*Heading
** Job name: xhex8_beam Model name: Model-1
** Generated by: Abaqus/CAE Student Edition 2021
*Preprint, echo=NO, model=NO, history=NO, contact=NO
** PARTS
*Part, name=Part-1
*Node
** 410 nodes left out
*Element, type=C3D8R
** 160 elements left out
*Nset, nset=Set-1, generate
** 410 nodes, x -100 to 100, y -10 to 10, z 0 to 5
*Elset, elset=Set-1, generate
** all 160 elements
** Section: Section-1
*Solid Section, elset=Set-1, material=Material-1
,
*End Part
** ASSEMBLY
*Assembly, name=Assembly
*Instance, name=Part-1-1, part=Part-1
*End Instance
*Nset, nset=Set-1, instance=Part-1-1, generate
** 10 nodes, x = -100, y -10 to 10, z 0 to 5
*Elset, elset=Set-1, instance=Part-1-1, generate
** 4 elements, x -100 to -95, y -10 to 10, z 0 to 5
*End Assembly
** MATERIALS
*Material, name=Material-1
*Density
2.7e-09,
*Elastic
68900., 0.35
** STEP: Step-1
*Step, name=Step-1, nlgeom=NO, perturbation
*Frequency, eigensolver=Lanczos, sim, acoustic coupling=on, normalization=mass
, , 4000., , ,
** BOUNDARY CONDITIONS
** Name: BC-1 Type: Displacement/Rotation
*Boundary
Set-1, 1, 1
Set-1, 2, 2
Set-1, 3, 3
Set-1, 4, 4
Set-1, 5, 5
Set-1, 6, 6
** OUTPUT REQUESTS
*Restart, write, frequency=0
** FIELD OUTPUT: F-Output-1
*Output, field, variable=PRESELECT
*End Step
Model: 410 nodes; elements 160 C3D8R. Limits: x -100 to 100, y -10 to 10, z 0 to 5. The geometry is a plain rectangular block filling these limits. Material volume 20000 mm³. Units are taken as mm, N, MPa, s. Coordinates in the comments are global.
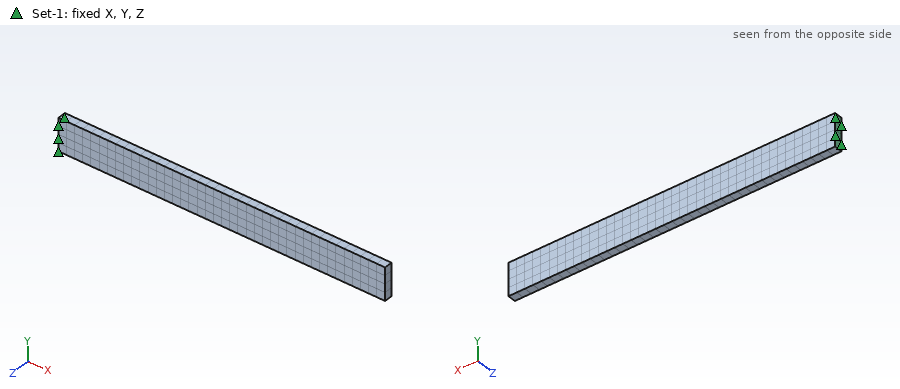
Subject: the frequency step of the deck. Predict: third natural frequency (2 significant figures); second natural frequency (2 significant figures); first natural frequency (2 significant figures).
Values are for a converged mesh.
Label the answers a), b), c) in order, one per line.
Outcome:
a) 640 Hz
b) 410 Hz
c) 100 Hz
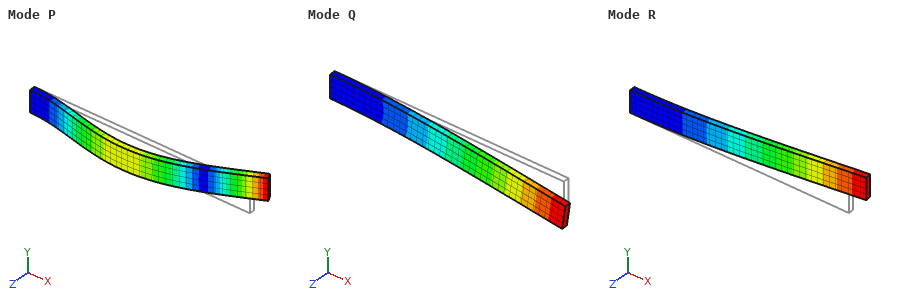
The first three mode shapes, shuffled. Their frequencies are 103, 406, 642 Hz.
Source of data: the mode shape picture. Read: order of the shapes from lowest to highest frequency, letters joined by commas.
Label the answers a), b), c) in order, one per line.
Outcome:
a) R, Q, P
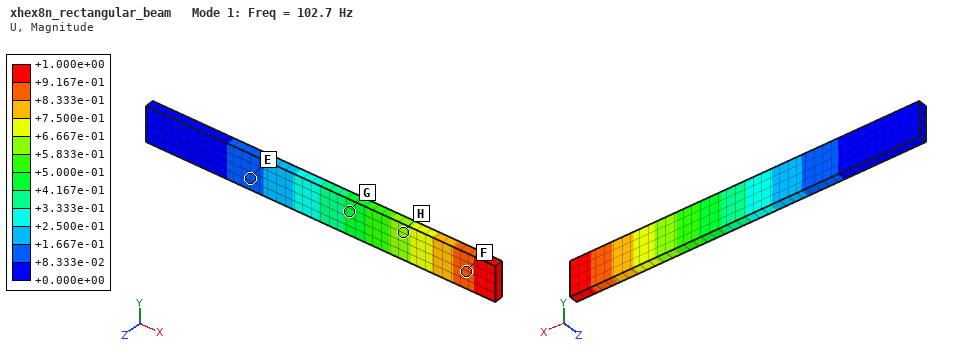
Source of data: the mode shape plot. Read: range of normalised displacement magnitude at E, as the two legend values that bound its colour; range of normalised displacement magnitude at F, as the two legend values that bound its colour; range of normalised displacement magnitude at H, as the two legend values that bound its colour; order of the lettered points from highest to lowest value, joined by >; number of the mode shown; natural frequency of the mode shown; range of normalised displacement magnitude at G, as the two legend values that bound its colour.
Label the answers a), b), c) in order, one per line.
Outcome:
a) +8.333e-02 to +1.667e-01
b) +8.333e-01 to +9.167e-01
c) +5.833e-01 to +6.667e-01
d) F > H > G > E
e) 1
f) 102.7 Hz
g) +4.167e-01 to +5.000e-01
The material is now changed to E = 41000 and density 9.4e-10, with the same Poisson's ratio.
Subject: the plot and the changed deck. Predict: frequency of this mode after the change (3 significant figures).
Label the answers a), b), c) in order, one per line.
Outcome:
a) 134 Hz
